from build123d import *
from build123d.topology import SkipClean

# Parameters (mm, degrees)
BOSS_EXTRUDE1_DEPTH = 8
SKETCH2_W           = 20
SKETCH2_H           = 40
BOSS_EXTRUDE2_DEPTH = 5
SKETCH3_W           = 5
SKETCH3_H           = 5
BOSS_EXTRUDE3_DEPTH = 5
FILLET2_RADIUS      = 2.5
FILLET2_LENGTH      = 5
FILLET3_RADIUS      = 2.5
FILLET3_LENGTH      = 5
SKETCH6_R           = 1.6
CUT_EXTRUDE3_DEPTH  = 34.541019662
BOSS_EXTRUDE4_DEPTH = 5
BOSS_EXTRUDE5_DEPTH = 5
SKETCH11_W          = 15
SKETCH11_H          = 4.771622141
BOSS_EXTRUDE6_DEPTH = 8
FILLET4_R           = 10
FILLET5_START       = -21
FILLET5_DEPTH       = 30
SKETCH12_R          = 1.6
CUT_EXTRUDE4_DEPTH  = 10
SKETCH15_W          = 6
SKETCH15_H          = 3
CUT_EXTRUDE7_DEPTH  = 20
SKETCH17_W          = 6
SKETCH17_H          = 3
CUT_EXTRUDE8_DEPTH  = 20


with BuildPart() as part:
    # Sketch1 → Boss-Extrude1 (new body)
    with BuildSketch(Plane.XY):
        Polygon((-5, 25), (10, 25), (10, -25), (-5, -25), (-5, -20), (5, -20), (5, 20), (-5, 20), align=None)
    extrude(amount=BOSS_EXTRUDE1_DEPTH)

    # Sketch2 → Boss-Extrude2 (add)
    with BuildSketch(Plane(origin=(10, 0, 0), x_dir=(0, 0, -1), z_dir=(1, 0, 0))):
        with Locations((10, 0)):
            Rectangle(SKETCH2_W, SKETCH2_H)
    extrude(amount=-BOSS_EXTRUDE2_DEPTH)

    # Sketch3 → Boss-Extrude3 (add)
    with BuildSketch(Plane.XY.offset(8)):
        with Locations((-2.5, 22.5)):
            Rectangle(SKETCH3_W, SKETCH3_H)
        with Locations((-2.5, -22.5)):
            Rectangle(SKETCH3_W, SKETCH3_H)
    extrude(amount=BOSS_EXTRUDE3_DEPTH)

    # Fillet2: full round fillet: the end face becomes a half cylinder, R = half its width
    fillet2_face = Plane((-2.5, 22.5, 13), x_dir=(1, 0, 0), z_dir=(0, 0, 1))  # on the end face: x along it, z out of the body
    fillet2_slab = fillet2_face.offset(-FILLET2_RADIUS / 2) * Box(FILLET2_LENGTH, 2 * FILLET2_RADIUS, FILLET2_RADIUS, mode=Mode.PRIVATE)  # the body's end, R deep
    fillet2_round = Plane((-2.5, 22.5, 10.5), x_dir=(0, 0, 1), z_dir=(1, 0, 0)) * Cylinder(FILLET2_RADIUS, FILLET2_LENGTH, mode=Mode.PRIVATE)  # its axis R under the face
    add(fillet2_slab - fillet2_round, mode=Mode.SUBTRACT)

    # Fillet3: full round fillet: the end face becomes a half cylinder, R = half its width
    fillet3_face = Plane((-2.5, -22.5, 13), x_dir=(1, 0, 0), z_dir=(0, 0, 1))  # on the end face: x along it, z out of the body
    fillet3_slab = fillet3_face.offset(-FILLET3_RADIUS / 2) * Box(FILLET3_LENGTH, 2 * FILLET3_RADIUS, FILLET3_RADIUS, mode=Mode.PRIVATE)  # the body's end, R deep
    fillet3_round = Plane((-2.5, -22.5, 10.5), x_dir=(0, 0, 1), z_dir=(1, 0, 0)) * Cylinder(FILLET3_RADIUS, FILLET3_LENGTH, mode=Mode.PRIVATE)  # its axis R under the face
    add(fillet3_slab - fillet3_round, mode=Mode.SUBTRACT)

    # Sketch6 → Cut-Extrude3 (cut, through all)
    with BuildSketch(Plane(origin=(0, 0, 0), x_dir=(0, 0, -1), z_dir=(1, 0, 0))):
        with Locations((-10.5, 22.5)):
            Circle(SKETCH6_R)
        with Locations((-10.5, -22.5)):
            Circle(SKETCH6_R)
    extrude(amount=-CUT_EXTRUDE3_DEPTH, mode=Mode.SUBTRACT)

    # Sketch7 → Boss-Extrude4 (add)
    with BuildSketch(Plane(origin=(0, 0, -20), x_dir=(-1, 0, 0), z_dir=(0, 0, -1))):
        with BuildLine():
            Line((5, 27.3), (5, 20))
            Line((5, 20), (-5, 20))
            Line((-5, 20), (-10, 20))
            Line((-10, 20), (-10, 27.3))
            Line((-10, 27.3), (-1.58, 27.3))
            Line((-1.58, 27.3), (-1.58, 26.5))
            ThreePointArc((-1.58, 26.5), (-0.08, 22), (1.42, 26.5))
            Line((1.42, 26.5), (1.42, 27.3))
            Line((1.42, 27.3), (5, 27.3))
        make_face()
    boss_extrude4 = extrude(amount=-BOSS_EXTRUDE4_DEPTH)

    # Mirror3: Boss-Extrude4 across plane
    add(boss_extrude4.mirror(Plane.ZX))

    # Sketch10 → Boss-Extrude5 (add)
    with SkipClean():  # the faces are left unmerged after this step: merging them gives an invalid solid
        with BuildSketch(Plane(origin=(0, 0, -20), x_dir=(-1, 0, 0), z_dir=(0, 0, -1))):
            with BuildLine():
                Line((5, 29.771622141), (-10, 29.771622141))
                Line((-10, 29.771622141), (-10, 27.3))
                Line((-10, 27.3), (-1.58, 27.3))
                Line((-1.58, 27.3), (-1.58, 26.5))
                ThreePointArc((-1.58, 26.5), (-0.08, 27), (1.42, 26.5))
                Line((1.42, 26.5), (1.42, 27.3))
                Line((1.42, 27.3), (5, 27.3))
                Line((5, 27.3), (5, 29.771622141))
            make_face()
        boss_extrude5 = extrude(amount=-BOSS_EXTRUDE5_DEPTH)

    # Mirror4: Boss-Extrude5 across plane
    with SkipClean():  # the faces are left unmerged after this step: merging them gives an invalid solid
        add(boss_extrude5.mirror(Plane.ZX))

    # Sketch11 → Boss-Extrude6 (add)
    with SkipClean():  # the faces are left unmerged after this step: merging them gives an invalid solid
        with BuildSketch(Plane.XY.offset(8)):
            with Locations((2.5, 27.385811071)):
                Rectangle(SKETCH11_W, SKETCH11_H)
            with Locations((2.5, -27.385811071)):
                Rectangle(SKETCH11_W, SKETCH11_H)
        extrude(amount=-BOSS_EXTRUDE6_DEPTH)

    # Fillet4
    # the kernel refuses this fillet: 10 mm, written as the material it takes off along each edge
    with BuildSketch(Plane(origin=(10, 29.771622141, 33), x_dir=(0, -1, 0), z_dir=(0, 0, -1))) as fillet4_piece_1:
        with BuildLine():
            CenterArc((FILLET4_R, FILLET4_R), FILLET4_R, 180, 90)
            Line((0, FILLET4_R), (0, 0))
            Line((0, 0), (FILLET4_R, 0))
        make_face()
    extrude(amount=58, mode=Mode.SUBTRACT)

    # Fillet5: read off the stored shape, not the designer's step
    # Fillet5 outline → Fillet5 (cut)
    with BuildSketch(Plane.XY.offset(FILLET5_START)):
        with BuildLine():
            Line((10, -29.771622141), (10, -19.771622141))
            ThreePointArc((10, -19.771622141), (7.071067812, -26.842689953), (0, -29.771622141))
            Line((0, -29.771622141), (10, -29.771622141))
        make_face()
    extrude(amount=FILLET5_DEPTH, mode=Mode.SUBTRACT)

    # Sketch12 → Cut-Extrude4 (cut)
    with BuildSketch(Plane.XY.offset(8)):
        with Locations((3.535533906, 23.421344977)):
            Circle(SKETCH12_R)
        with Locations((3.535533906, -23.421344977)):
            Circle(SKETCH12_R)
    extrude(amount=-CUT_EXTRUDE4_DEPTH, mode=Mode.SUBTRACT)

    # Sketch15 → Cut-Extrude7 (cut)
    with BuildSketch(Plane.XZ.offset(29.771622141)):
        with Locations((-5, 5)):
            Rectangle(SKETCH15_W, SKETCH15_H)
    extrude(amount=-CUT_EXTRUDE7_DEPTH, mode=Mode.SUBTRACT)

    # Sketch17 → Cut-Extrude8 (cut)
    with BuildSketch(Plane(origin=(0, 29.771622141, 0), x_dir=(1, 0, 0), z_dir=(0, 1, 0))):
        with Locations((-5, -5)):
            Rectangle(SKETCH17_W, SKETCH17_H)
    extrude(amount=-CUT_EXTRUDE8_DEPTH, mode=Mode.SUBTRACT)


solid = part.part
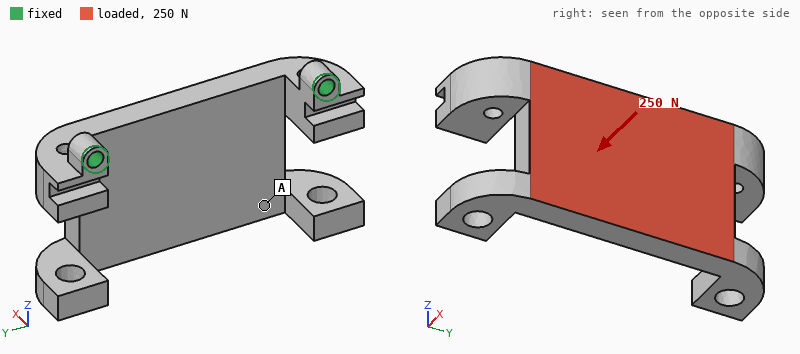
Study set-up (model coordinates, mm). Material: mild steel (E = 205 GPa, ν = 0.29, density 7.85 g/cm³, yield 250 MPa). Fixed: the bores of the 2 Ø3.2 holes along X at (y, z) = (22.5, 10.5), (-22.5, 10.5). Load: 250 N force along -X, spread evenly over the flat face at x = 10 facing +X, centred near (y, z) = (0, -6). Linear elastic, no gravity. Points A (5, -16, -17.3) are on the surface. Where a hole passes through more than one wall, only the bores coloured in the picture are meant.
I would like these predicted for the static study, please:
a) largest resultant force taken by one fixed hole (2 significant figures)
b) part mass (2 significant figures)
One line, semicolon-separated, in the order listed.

150 N; 67 g
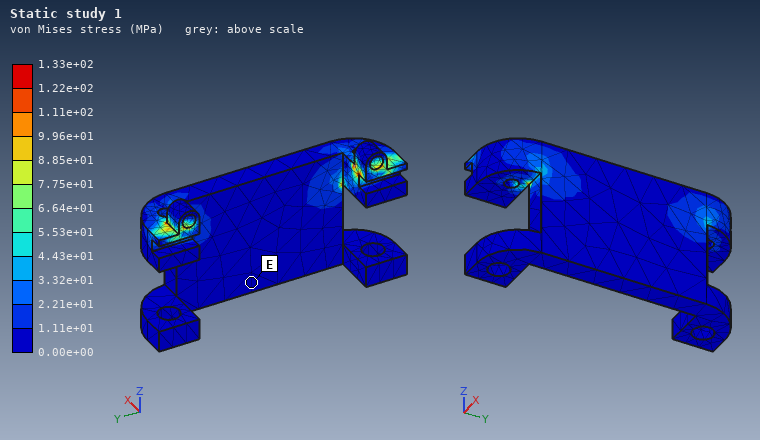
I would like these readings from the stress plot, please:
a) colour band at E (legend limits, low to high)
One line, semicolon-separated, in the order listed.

0.00e+00 to 1.11e+01 MPa
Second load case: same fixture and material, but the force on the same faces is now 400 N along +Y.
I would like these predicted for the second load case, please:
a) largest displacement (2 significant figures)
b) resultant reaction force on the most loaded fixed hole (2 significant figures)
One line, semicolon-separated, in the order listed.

9.8 µm; 240 N
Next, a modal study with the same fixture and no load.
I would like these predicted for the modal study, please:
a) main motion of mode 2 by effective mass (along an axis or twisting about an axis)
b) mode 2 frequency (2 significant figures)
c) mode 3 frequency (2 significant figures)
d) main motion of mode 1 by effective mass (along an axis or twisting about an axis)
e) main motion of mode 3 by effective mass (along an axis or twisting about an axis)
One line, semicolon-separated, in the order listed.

along Y; 3500 Hz; 5800 Hz; along X; along Z
